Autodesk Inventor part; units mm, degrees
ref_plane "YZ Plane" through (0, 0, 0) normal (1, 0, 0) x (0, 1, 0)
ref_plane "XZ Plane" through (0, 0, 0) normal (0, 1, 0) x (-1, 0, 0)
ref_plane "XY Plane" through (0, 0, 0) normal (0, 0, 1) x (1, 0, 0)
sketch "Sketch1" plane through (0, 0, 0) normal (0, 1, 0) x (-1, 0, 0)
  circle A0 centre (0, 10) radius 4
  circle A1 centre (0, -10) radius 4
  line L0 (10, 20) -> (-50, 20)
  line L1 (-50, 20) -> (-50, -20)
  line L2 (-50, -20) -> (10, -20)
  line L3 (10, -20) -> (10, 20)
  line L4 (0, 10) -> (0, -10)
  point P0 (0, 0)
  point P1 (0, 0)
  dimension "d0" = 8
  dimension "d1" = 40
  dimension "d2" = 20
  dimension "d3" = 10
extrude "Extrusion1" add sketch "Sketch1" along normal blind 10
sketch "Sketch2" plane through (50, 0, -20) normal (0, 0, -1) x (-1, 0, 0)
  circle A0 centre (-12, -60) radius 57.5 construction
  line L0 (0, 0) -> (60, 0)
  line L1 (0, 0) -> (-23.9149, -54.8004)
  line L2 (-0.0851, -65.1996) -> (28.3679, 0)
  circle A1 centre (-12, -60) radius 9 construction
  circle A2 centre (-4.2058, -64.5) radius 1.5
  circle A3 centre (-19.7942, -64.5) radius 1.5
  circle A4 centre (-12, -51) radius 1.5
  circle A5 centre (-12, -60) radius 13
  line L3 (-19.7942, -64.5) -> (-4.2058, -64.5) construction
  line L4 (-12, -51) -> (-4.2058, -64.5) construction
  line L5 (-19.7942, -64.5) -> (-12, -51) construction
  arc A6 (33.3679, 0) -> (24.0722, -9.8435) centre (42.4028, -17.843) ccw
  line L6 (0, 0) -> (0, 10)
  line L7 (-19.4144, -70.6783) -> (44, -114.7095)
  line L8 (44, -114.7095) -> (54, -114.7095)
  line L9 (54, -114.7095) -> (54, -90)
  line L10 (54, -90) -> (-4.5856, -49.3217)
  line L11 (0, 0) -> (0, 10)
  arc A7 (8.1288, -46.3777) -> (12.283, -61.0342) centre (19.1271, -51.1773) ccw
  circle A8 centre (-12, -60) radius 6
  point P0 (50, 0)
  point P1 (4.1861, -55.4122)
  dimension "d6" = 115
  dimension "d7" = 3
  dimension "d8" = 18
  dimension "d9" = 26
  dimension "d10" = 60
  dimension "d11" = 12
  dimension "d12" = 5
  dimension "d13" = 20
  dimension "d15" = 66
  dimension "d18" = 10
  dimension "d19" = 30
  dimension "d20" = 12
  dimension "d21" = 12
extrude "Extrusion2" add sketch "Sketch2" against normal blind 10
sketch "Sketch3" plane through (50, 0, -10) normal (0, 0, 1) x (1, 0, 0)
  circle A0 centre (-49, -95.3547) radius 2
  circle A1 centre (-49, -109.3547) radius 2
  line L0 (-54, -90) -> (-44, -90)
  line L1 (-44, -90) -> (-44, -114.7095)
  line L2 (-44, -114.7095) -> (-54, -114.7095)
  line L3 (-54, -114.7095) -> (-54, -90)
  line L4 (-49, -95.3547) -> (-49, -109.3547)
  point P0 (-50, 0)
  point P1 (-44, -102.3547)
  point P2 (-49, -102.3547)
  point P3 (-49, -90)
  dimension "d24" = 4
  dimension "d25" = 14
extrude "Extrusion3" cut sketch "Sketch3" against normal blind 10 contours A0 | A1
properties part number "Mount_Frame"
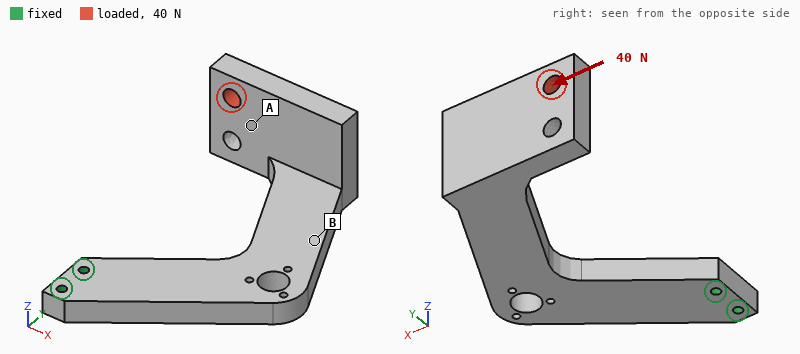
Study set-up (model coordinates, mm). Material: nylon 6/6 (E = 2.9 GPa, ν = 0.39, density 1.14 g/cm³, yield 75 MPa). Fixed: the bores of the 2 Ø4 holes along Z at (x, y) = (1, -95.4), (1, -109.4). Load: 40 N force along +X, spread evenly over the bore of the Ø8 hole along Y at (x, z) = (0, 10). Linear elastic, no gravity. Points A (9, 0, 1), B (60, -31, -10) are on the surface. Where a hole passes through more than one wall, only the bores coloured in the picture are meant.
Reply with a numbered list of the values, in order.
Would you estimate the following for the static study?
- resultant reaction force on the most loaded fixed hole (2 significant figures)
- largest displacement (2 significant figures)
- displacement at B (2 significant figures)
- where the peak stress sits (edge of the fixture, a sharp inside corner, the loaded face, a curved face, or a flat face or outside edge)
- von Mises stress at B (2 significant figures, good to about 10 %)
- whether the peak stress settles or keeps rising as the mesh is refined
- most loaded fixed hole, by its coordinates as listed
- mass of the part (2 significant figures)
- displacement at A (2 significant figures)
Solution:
1. 290 N
2. 1.7 mm
3. 0.62 mm
4. edge of the fixture
5. 2.6 MPa
6. keeps rising
7. (1, -95.4)
8. 67 g
9. 1.1 mm
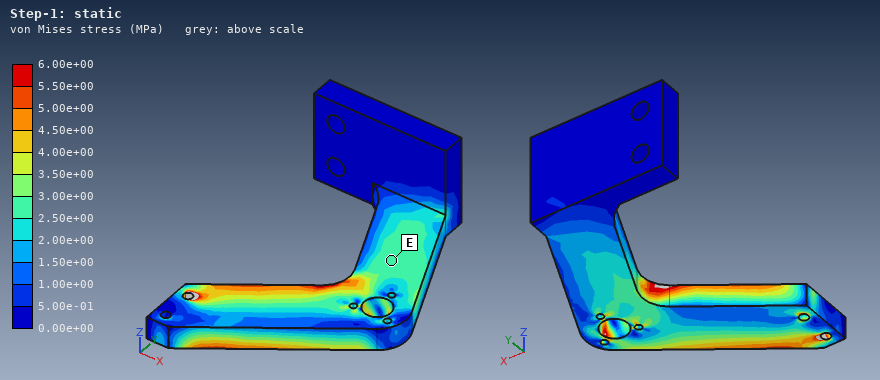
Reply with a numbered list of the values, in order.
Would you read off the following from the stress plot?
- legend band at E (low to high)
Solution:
1. 2.50e+00 to 3.00e+00 MPa
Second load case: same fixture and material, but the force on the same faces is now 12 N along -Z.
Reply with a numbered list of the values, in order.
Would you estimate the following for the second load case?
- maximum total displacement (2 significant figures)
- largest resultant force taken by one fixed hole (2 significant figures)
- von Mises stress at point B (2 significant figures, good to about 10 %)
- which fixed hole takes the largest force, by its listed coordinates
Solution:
1. 1.7 mm
2. 53 N
3. 1.5 MPa
4. (1, -95.4)
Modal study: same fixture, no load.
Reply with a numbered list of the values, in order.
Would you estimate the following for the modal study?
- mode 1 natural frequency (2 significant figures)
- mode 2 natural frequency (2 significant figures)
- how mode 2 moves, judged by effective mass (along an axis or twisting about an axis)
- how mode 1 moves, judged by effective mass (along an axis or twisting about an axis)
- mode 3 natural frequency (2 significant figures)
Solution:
1. 87 Hz
2. 180 Hz
3. along X
4. along Z
5. 270 Hz
